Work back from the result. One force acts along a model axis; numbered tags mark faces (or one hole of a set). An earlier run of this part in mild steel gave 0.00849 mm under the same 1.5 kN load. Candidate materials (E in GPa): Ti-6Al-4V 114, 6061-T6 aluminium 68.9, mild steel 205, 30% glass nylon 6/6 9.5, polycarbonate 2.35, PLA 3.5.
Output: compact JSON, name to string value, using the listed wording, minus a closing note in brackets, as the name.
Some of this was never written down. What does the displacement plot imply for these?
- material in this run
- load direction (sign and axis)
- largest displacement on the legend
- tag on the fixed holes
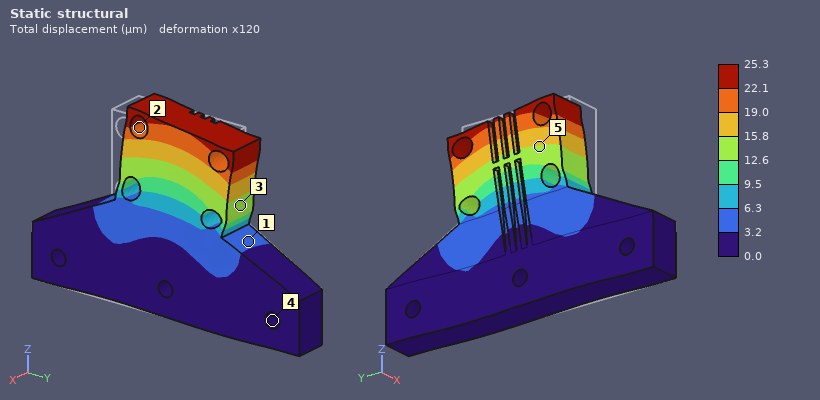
{"material in this run": "6061-T6 aluminium", "load direction": "+Y", "largest displacement on the legend": "25.3 µm", "tag on the fixed holes": "4"}
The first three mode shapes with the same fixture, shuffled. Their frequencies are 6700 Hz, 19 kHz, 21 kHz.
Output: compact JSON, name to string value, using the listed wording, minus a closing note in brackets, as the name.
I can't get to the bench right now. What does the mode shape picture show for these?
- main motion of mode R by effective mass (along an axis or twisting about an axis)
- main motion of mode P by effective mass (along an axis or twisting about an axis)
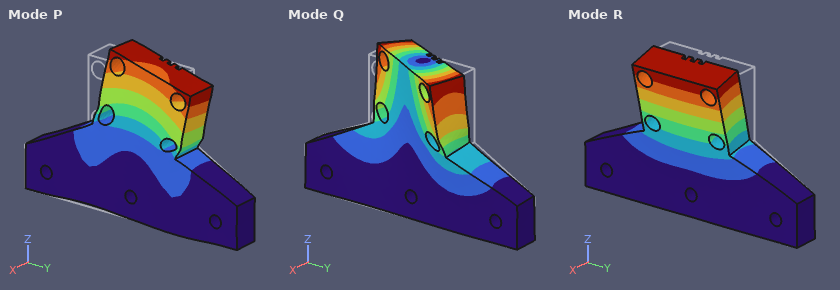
{"main motion of mode R by effective mass": "along X", "main motion of mode P by effective mass": "along Y"}
